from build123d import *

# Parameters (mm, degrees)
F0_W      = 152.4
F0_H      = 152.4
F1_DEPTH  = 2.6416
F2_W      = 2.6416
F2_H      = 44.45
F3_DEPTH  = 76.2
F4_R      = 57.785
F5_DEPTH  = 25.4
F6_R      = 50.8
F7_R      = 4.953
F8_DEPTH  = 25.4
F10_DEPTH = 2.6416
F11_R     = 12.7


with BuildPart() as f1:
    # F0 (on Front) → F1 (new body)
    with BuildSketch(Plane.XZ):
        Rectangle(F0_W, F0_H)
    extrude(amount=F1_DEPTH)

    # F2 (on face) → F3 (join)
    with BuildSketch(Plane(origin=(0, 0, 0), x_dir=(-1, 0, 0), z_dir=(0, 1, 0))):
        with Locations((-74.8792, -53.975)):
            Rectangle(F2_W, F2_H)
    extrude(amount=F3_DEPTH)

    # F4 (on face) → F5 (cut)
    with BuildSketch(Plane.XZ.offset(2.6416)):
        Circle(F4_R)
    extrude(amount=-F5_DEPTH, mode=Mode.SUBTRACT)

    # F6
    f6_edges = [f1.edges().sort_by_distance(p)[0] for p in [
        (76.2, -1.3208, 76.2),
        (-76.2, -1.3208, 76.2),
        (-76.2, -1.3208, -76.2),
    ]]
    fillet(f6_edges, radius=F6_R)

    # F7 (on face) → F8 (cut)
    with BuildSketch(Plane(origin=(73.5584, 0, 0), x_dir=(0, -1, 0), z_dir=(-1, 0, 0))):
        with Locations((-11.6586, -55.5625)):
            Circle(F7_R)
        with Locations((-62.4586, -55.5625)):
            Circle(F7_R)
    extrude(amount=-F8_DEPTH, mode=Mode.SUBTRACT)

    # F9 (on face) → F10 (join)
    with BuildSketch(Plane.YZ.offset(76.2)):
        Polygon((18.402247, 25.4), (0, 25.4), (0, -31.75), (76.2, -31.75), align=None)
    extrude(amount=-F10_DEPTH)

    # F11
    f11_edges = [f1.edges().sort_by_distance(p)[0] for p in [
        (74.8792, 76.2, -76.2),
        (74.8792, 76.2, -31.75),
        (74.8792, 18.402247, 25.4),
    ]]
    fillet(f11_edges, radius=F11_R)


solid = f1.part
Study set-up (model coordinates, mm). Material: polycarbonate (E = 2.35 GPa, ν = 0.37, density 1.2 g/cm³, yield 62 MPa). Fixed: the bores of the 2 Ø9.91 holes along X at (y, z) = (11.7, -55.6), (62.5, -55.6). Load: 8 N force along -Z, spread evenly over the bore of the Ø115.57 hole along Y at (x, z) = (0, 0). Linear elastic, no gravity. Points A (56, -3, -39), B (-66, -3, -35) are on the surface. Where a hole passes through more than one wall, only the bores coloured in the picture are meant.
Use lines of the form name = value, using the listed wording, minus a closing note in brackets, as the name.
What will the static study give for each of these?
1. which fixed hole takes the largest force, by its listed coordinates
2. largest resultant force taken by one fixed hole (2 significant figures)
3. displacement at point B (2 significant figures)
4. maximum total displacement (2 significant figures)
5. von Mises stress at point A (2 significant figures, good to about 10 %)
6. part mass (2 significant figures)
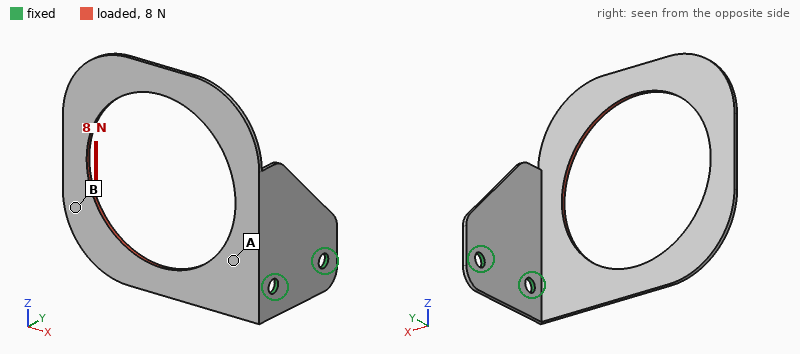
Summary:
which fixed hole takes the largest force, by its listed coordinates = (11.7, -55.6)
largest resultant force taken by one fixed hole = 8.7 N
displacement at point B = 2.1 mm
maximum total displacement = 2.8 mm
von Mises stress at point A = 0.97 MPa
part mass = 54 g
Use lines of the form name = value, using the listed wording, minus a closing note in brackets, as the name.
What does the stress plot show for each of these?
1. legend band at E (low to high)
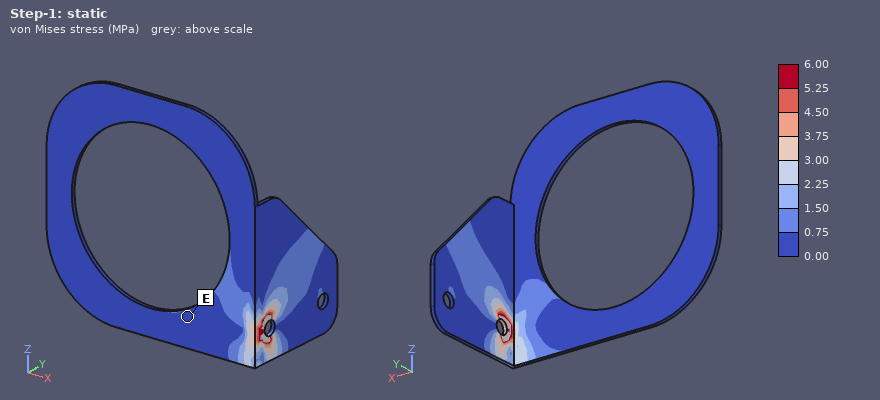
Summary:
legend band at E = 0.00 to 0.75 MPa
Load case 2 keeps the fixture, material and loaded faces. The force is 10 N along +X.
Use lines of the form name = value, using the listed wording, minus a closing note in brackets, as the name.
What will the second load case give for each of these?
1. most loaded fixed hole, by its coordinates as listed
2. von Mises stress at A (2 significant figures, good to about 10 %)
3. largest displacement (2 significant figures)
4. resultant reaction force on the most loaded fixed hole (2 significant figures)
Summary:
most loaded fixed hole, by its coordinates as listed = (11.7, -55.6)
von Mises stress at A = 1.0 MPa
largest displacement = 2.7 mm
resultant reaction force on the most loaded fixed hole = 11 N
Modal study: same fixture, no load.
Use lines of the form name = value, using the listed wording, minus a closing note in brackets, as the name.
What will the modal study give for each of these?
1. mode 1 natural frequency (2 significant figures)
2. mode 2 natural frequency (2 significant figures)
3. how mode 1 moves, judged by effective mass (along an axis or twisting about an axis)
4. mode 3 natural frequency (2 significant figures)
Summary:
mode 1 natural frequency = 18 Hz
mode 2 natural frequency = 45 Hz
how mode 1 moves, judged by effective mass = along Y
mode 3 natural frequency = 49 Hz
